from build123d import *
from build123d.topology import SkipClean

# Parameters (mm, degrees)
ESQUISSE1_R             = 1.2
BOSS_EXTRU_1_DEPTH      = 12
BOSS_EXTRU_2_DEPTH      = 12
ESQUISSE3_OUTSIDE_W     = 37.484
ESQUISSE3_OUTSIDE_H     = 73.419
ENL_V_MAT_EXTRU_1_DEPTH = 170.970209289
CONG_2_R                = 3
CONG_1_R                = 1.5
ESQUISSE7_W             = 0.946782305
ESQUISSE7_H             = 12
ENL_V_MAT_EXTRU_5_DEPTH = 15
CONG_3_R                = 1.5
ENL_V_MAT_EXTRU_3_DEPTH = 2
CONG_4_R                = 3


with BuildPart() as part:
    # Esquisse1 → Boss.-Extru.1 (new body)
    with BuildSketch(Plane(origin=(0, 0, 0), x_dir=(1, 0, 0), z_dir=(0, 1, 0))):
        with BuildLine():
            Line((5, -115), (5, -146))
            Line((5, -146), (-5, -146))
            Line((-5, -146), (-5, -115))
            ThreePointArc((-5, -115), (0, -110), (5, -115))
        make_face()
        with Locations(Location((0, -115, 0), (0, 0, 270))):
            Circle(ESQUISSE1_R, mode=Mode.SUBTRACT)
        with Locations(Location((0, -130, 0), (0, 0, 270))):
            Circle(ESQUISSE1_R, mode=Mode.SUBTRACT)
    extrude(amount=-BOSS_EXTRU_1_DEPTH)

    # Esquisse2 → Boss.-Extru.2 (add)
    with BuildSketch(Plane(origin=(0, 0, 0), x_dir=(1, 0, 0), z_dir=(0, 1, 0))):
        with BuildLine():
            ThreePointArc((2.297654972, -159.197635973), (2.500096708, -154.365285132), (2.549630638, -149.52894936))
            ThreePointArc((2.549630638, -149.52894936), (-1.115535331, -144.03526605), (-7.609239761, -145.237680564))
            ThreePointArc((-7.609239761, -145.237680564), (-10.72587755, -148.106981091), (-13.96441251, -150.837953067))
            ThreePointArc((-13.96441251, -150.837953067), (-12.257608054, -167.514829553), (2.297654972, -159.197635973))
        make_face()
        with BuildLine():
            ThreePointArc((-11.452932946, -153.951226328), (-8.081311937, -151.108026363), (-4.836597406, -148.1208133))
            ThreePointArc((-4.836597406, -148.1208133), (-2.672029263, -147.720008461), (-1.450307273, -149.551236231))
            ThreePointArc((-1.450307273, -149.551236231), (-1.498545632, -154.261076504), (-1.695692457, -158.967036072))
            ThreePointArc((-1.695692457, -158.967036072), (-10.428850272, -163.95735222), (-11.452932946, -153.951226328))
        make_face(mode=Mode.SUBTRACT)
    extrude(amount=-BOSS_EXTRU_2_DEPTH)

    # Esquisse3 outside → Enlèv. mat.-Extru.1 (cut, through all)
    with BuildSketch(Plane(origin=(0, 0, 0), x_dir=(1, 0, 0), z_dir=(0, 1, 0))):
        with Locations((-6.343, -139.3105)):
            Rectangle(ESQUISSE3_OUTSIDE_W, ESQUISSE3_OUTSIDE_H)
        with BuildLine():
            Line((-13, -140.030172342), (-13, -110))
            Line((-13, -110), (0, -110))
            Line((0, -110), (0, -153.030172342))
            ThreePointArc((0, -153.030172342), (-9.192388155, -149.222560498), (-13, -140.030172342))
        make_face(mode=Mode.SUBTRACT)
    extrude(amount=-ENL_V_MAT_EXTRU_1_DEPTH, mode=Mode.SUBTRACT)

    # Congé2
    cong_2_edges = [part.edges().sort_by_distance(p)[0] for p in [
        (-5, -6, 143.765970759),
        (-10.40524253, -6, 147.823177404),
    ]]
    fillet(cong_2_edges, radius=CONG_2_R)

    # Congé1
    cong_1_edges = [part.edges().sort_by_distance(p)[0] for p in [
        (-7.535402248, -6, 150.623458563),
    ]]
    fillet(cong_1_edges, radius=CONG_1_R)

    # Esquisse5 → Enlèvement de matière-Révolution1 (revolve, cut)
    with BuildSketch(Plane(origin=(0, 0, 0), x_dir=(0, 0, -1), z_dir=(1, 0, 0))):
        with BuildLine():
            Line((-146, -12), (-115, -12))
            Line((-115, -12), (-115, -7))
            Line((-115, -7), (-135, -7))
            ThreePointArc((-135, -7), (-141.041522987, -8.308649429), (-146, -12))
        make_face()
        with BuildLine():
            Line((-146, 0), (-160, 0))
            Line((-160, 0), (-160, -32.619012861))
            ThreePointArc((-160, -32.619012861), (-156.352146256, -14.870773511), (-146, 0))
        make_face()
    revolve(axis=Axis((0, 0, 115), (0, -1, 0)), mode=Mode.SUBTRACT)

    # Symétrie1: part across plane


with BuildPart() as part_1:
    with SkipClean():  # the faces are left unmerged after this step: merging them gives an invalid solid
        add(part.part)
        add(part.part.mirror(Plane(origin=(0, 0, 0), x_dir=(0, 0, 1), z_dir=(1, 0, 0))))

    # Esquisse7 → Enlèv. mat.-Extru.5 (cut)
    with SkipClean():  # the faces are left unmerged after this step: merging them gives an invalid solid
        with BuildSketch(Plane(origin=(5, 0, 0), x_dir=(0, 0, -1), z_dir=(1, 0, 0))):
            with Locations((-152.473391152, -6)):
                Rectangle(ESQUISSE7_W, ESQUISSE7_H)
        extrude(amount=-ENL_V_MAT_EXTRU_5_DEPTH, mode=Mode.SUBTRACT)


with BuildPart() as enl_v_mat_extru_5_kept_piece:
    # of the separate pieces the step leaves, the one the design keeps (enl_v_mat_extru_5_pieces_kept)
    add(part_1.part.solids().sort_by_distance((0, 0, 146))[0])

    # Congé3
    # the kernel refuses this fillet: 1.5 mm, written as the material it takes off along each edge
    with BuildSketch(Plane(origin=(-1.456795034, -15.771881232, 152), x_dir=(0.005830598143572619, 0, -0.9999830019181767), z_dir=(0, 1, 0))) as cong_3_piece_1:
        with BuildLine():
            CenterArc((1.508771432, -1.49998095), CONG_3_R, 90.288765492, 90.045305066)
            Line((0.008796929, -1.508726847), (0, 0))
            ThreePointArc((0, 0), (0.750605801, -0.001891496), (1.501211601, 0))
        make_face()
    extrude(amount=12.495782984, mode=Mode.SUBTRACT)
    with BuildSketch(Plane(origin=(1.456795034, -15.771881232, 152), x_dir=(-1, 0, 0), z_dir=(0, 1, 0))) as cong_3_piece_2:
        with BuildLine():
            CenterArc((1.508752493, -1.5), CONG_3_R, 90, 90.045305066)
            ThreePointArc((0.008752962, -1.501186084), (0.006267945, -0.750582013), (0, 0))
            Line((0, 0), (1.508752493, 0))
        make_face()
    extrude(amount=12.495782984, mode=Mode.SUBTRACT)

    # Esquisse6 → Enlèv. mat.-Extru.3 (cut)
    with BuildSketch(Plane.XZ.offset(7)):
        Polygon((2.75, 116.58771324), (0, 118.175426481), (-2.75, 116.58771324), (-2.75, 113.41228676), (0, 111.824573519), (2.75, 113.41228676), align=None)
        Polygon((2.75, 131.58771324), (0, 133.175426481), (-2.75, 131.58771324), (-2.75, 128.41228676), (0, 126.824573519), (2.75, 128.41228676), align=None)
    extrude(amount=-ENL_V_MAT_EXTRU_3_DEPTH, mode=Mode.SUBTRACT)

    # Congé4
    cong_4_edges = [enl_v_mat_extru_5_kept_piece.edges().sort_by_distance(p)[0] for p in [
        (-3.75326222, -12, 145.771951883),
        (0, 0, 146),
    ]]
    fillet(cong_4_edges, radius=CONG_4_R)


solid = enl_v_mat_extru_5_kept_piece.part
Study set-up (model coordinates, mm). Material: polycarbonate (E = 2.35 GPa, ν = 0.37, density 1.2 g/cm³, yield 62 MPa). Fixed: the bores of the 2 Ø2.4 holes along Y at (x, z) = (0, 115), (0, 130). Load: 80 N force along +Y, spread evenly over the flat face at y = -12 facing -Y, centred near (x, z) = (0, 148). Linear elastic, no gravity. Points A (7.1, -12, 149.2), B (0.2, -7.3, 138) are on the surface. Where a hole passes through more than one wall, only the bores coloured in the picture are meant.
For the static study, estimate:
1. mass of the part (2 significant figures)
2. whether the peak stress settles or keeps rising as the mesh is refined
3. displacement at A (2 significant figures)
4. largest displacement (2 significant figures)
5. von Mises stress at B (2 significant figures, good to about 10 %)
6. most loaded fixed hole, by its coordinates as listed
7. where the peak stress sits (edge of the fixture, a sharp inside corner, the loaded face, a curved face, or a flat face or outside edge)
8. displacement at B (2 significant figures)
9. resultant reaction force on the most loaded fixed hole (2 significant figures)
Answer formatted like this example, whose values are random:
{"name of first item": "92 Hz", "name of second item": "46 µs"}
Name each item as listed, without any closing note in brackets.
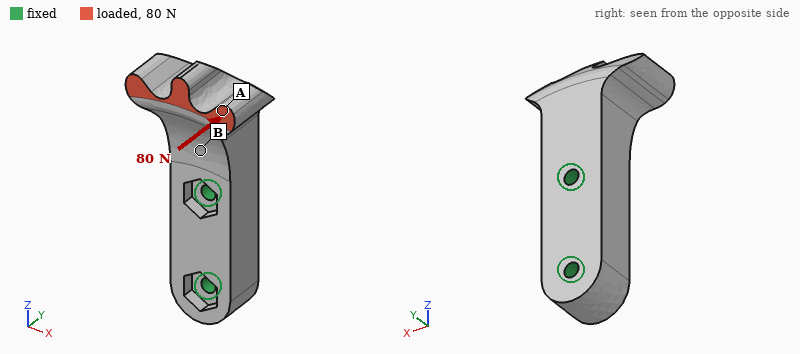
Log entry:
{"mass of the part": "3.8 g", "whether the peak stress settles or keeps rising as the mesh is refined": "keeps rising", "displacement at A": "0.47 mm", "largest displacement": "0.53 mm", "von Mises stress at B": "8.4 MPa", "most loaded fixed hole, by its coordinates as listed": "(0, 130)", "where the peak stress sits": "edge of the fixture", "displacement at B": "0.16 mm", "resultant reaction force on the most loaded fixed hole": "130 N"}
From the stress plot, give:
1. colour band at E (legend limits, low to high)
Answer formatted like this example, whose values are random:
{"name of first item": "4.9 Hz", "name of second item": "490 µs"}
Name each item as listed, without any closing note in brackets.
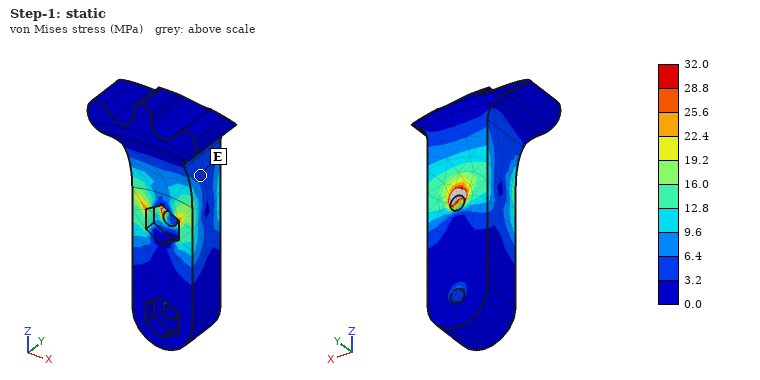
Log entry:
{"colour band at E": "3.2 to 6.4 MPa"}
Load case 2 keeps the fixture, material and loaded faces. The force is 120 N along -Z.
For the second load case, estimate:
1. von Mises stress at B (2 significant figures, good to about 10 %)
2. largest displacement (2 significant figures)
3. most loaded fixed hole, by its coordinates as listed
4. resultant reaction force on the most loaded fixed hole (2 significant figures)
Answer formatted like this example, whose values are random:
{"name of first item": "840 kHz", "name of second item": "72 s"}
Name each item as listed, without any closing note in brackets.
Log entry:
{"von Mises stress at B": "13 MPa", "largest displacement": "0.50 mm", "most loaded fixed hole, by its coordinates as listed": "(0, 130)", "resultant reaction force on the most loaded fixed hole": "80 N"}
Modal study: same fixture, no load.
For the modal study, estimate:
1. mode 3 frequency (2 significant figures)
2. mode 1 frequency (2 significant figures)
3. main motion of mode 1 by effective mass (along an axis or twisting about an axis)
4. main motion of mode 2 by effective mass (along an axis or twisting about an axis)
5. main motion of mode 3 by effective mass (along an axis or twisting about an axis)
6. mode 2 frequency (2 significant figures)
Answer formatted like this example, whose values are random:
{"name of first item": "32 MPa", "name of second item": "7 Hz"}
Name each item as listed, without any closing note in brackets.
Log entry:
{"mode 3 frequency": "4600 Hz", "mode 1 frequency": "2100 Hz", "main motion of mode 1 by effective mass": "along Y", "main motion of mode 2 by effective mass": "along X", "main motion of mode 3 by effective mass": "twisting about Z", "mode 2 frequency": "2500 Hz"}
